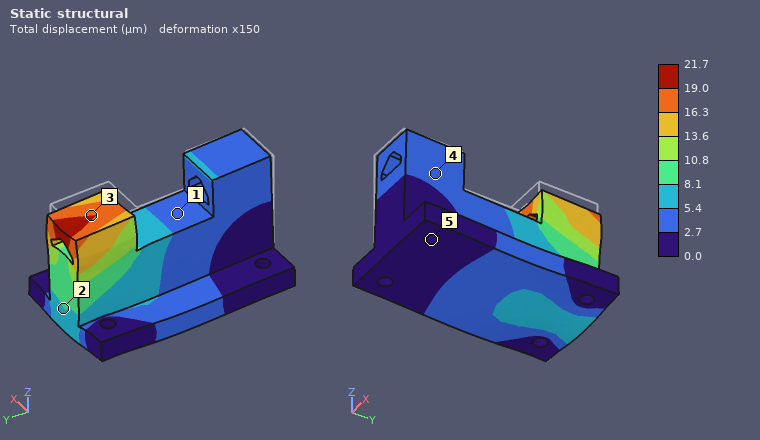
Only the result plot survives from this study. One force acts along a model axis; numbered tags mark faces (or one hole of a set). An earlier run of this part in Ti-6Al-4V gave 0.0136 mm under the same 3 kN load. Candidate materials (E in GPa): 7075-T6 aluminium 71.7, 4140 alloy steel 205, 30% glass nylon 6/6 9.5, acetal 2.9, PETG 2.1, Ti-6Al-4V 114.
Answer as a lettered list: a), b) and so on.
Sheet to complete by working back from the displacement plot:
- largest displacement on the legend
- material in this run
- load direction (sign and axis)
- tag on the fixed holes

a) 21.7 µm
b) 7075-T6 aluminium
c) -Z
d) 5
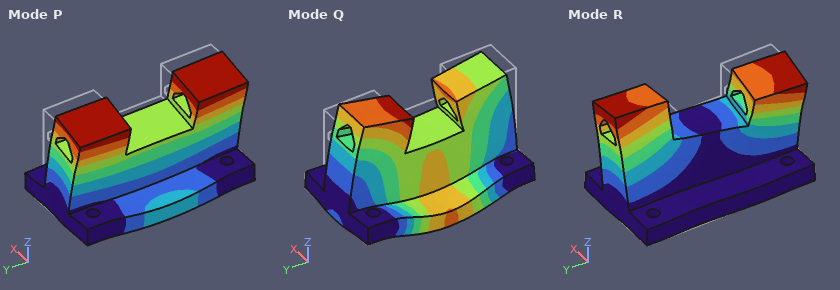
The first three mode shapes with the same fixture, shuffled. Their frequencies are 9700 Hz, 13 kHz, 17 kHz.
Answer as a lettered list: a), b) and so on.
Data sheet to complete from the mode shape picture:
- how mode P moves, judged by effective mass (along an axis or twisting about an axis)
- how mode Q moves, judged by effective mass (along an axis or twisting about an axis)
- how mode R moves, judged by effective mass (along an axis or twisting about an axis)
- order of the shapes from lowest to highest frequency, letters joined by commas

a) along X
b) along Z
c) twisting about Z
d) P, R, Q
